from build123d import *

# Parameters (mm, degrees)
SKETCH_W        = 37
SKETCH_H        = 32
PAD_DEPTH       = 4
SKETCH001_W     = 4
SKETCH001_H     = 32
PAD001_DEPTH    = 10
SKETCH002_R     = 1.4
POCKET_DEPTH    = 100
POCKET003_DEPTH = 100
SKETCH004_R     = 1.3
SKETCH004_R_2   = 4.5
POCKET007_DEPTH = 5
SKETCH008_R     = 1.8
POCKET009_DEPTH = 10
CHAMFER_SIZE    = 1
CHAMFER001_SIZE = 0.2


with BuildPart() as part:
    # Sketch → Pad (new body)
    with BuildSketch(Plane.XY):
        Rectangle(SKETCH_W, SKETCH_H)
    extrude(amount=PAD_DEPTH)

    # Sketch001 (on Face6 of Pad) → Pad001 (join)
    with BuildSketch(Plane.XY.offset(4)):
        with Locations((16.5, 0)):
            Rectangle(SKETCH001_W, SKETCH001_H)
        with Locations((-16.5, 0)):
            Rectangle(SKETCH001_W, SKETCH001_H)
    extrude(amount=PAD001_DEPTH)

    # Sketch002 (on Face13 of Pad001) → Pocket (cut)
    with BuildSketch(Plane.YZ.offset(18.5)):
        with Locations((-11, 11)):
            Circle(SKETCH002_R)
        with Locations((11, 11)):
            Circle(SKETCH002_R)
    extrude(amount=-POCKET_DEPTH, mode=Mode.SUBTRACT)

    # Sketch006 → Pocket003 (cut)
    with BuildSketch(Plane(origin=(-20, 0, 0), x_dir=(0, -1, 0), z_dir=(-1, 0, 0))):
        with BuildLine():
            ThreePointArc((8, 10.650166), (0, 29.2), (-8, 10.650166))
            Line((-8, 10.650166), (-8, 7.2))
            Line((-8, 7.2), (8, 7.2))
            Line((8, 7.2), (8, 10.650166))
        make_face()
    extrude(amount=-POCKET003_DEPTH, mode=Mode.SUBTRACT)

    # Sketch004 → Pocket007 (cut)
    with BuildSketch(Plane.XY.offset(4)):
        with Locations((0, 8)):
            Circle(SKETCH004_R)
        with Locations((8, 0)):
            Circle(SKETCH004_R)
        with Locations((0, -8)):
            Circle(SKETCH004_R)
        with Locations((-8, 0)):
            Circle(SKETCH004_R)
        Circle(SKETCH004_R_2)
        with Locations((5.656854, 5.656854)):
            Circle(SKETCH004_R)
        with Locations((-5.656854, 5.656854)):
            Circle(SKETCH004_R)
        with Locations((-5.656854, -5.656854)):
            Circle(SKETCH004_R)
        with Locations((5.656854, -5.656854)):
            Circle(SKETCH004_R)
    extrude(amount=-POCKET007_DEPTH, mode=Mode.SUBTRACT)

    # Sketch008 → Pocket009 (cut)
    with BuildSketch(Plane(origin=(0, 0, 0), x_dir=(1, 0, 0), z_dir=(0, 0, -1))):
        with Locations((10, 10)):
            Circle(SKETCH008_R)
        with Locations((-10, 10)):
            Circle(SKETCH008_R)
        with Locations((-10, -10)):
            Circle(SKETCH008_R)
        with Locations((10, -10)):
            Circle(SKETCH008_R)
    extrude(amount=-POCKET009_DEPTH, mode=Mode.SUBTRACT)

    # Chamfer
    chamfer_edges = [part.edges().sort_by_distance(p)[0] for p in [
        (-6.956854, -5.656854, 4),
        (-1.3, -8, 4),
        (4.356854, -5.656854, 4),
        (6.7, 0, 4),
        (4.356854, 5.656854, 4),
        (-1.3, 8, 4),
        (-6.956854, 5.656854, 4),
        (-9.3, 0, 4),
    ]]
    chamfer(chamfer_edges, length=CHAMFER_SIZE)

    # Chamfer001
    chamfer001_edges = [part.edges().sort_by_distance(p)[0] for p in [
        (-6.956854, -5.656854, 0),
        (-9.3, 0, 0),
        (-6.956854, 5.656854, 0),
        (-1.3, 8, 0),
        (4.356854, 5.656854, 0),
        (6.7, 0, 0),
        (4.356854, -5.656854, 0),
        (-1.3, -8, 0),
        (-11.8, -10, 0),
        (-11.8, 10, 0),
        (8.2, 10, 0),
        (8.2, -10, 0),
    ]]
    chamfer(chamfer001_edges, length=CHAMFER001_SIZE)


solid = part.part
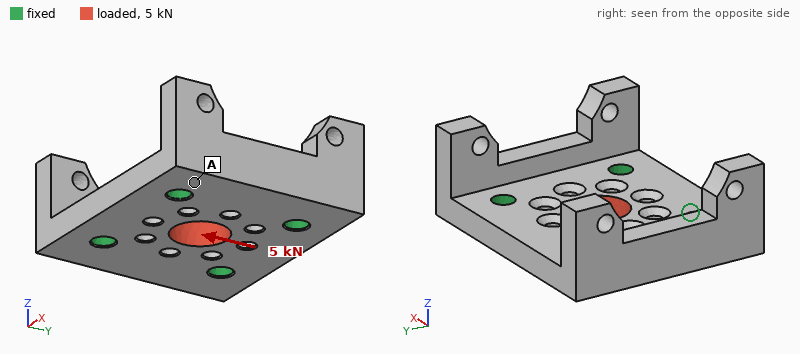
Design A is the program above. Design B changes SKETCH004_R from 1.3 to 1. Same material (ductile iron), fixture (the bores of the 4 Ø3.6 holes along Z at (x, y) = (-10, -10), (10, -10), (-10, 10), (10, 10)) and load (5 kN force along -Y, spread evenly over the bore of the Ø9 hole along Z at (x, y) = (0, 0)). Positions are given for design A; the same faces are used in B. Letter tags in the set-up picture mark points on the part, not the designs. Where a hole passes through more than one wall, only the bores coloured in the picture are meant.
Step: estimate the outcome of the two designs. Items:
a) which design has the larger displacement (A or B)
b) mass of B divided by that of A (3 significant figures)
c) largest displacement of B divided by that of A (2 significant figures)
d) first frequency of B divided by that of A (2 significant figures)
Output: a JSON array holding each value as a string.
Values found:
["A", "1.01", "0.90", "1.0"]
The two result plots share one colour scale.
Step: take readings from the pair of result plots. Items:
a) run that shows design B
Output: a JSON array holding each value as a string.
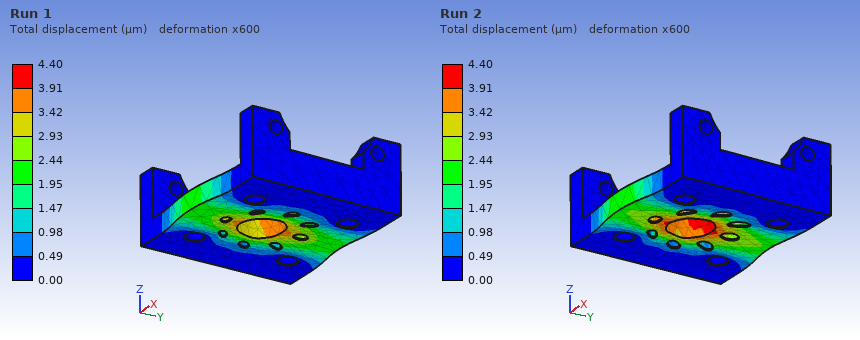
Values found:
["Run 1"]
